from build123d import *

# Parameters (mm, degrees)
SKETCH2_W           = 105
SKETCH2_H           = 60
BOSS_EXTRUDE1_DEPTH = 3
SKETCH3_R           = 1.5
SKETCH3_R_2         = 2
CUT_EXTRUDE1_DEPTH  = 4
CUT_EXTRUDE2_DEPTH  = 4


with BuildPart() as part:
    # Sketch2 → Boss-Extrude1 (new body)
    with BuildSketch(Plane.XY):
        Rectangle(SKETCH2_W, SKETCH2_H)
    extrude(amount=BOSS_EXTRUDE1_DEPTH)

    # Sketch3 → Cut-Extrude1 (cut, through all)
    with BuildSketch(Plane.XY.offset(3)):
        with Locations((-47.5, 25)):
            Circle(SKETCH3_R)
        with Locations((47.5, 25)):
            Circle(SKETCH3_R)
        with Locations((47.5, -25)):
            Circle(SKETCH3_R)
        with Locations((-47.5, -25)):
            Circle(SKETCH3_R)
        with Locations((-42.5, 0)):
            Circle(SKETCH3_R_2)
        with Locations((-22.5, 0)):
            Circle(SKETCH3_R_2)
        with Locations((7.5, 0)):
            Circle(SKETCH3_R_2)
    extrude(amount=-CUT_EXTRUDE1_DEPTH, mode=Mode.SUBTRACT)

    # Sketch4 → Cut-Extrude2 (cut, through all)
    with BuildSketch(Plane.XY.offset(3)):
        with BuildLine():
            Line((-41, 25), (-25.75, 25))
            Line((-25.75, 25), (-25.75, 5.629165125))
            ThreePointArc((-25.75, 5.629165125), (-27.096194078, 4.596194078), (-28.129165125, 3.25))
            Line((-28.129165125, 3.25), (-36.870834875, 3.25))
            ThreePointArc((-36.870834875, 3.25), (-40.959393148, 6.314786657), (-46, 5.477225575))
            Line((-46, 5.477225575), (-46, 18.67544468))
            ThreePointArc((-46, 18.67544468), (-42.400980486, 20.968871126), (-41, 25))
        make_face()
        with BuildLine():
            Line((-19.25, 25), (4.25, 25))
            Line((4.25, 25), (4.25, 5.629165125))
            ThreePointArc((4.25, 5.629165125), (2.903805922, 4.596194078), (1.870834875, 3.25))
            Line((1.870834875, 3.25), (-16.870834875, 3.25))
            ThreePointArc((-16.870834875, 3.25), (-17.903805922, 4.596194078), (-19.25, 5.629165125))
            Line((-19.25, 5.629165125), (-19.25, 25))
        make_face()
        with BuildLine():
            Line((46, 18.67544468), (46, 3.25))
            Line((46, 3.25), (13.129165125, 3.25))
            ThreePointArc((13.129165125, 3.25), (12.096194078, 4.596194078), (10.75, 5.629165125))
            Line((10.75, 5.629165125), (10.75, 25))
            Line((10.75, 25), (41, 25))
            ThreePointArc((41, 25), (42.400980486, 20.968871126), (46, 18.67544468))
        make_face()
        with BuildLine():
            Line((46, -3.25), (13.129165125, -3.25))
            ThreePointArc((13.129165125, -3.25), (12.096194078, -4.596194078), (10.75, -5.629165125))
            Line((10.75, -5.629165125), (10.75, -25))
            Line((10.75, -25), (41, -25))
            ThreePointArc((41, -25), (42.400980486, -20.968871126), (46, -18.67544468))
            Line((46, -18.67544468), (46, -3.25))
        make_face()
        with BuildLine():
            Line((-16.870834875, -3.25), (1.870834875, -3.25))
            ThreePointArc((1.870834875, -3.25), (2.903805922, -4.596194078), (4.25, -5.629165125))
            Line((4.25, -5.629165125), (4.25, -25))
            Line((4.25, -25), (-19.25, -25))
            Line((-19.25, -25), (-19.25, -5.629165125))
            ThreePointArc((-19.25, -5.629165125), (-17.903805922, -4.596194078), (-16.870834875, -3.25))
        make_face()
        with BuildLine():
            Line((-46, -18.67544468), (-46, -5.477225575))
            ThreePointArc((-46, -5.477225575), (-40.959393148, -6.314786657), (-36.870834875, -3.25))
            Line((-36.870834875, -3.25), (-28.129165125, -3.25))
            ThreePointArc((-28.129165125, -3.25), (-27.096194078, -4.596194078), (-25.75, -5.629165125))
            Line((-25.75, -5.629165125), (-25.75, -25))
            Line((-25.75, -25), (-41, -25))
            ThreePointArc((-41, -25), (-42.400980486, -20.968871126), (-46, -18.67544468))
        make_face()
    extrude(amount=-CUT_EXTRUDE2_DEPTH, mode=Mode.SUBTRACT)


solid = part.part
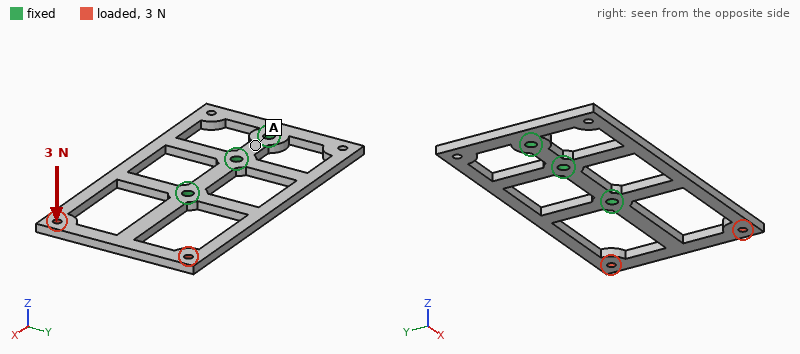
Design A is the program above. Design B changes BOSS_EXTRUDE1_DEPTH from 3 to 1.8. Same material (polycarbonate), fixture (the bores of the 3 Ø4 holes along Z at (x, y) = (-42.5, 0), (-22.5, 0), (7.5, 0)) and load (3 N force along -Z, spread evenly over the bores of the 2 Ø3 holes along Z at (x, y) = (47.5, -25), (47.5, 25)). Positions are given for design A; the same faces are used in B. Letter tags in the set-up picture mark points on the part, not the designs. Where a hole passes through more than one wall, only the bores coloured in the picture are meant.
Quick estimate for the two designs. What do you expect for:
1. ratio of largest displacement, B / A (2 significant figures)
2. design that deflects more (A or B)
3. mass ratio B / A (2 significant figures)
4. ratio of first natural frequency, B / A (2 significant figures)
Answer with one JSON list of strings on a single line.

["4.5", "B", "0.60", "0.61"]
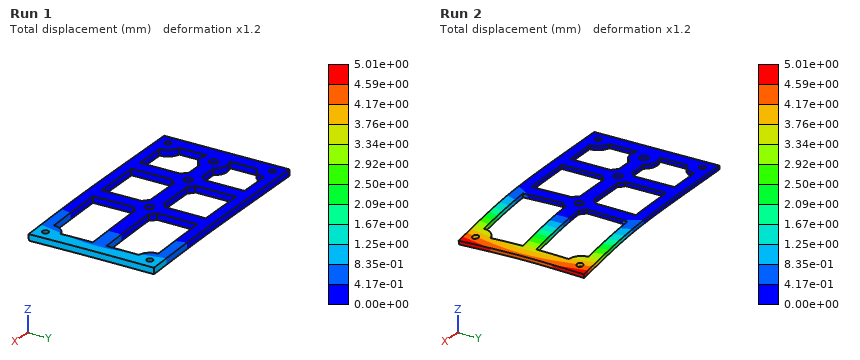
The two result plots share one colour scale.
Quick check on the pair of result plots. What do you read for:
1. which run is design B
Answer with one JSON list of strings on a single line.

["Run 2"]
